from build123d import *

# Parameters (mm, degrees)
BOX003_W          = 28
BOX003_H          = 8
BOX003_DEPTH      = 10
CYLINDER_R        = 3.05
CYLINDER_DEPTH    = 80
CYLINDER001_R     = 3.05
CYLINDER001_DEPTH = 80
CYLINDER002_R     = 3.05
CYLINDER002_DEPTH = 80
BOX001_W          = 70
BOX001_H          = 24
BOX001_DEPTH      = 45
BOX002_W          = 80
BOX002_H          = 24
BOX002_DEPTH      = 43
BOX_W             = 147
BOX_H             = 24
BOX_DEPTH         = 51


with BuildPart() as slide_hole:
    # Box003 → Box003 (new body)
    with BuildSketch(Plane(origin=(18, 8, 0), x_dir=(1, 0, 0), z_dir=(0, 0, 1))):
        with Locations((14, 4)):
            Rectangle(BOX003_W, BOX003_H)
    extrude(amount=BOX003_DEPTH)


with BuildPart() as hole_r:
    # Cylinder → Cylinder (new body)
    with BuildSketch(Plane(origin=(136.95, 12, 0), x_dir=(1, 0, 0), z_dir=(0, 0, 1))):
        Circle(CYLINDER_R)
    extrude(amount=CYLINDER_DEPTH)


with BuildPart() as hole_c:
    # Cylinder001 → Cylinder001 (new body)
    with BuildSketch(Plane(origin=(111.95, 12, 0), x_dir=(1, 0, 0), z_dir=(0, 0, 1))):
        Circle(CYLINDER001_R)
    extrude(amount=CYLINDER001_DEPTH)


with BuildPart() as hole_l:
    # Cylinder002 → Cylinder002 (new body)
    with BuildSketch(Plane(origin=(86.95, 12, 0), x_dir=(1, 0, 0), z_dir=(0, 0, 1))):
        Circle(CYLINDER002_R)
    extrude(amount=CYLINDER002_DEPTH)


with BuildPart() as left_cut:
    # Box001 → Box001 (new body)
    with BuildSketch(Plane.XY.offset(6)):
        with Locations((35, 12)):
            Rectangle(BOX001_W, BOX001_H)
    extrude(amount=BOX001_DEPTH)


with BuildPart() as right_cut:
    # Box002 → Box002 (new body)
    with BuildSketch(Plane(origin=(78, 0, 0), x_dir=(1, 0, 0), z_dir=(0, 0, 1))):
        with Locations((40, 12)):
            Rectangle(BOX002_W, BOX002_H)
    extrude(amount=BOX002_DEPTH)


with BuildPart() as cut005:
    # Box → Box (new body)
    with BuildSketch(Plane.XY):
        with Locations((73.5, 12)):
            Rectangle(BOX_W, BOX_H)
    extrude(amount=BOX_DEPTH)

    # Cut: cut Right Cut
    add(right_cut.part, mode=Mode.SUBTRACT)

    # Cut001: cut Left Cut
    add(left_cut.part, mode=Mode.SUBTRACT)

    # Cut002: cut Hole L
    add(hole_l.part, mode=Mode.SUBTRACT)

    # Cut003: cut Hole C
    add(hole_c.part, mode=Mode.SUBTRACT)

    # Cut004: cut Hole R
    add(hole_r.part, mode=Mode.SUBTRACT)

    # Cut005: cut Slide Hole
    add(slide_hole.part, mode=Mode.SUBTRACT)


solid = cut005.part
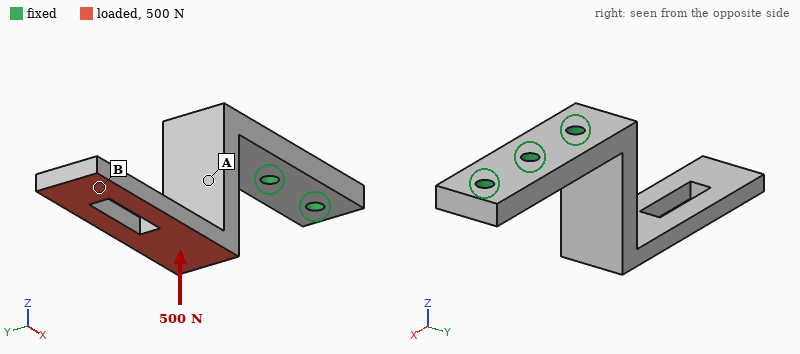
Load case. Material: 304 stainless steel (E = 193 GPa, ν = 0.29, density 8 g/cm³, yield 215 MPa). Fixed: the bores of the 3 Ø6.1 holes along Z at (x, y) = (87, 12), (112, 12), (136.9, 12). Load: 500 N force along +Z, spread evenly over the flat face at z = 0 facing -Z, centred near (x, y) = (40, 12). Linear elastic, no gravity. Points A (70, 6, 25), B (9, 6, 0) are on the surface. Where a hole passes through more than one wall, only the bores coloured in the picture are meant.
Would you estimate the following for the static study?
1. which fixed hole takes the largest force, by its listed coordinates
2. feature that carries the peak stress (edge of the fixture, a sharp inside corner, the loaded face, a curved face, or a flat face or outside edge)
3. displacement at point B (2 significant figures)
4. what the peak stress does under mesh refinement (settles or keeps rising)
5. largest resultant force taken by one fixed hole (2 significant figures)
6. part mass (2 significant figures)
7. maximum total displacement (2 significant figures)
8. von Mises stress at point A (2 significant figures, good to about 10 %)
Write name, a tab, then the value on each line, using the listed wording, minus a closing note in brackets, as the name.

which fixed hole takes the largest force, by its listed coordinates	(87, 12)
feature that carries the peak stress	edge of the fixture
displacement at point B	0.57 mm
what the peak stress does under mesh refinement	keeps rising
largest resultant force taken by one fixed hole	700 N
part mass	250 g
maximum total displacement	0.66 mm
von Mises stress at point A	68 MPa
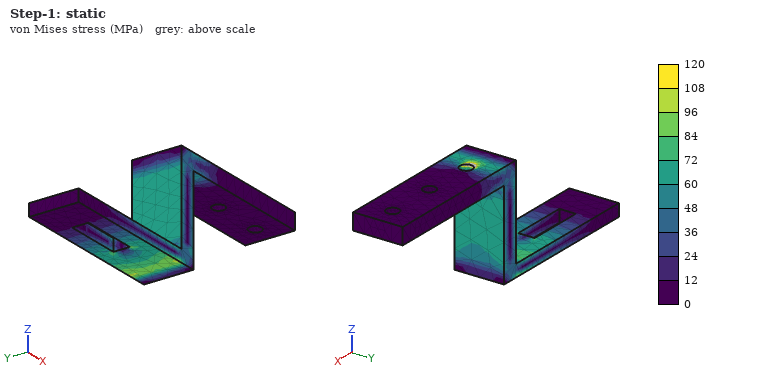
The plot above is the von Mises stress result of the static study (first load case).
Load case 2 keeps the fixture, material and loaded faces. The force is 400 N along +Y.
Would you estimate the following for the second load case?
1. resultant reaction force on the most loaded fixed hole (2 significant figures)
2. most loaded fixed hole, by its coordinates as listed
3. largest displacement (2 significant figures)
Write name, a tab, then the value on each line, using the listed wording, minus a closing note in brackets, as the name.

resultant reaction force on the most loaded fixed hole	830 N
most loaded fixed hole, by its coordinates as listed	(87, 12)
largest displacement	0.21 mm
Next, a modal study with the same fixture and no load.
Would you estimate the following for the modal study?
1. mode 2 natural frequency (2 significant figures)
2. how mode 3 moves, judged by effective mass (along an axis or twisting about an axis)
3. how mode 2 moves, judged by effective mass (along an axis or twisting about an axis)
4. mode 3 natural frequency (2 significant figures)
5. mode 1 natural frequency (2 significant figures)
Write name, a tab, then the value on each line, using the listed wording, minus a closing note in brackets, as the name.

mode 2 natural frequency	930 Hz
how mode 3 moves, judged by effective mass	along X
how mode 2 moves, judged by effective mass	along Y
mode 3 natural frequency	1500 Hz
mode 1 natural frequency	560 Hz
